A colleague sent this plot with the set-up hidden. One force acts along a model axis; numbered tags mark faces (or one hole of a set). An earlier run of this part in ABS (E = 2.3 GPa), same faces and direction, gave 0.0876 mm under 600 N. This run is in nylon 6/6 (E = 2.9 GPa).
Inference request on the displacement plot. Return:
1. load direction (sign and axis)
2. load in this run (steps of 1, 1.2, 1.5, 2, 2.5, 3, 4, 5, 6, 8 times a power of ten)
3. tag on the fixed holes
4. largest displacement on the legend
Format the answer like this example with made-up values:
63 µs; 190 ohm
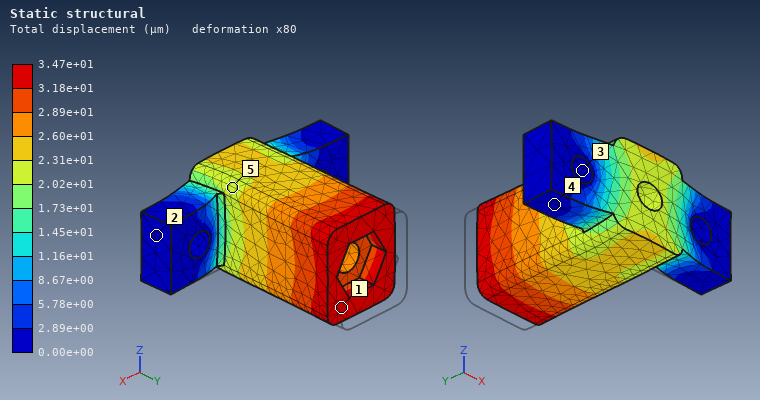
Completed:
-Y; 300 N; 3; 3.47e+01 µm
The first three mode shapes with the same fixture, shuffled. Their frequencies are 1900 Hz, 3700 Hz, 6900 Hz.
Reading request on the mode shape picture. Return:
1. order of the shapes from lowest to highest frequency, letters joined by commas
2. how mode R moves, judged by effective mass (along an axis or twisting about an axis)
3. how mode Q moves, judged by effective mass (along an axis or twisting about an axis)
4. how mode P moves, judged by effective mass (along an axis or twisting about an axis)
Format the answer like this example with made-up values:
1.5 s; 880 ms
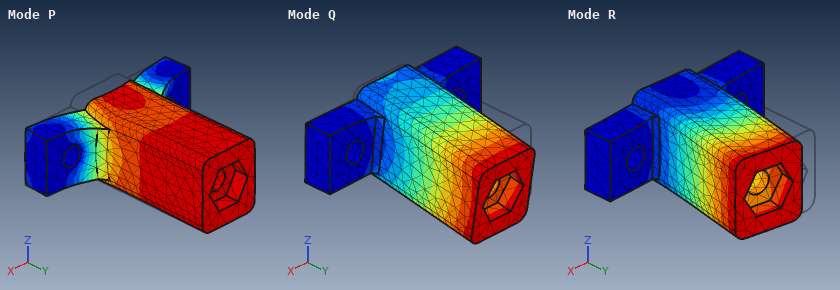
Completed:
Q, R, P; along X; along Z; along Y
